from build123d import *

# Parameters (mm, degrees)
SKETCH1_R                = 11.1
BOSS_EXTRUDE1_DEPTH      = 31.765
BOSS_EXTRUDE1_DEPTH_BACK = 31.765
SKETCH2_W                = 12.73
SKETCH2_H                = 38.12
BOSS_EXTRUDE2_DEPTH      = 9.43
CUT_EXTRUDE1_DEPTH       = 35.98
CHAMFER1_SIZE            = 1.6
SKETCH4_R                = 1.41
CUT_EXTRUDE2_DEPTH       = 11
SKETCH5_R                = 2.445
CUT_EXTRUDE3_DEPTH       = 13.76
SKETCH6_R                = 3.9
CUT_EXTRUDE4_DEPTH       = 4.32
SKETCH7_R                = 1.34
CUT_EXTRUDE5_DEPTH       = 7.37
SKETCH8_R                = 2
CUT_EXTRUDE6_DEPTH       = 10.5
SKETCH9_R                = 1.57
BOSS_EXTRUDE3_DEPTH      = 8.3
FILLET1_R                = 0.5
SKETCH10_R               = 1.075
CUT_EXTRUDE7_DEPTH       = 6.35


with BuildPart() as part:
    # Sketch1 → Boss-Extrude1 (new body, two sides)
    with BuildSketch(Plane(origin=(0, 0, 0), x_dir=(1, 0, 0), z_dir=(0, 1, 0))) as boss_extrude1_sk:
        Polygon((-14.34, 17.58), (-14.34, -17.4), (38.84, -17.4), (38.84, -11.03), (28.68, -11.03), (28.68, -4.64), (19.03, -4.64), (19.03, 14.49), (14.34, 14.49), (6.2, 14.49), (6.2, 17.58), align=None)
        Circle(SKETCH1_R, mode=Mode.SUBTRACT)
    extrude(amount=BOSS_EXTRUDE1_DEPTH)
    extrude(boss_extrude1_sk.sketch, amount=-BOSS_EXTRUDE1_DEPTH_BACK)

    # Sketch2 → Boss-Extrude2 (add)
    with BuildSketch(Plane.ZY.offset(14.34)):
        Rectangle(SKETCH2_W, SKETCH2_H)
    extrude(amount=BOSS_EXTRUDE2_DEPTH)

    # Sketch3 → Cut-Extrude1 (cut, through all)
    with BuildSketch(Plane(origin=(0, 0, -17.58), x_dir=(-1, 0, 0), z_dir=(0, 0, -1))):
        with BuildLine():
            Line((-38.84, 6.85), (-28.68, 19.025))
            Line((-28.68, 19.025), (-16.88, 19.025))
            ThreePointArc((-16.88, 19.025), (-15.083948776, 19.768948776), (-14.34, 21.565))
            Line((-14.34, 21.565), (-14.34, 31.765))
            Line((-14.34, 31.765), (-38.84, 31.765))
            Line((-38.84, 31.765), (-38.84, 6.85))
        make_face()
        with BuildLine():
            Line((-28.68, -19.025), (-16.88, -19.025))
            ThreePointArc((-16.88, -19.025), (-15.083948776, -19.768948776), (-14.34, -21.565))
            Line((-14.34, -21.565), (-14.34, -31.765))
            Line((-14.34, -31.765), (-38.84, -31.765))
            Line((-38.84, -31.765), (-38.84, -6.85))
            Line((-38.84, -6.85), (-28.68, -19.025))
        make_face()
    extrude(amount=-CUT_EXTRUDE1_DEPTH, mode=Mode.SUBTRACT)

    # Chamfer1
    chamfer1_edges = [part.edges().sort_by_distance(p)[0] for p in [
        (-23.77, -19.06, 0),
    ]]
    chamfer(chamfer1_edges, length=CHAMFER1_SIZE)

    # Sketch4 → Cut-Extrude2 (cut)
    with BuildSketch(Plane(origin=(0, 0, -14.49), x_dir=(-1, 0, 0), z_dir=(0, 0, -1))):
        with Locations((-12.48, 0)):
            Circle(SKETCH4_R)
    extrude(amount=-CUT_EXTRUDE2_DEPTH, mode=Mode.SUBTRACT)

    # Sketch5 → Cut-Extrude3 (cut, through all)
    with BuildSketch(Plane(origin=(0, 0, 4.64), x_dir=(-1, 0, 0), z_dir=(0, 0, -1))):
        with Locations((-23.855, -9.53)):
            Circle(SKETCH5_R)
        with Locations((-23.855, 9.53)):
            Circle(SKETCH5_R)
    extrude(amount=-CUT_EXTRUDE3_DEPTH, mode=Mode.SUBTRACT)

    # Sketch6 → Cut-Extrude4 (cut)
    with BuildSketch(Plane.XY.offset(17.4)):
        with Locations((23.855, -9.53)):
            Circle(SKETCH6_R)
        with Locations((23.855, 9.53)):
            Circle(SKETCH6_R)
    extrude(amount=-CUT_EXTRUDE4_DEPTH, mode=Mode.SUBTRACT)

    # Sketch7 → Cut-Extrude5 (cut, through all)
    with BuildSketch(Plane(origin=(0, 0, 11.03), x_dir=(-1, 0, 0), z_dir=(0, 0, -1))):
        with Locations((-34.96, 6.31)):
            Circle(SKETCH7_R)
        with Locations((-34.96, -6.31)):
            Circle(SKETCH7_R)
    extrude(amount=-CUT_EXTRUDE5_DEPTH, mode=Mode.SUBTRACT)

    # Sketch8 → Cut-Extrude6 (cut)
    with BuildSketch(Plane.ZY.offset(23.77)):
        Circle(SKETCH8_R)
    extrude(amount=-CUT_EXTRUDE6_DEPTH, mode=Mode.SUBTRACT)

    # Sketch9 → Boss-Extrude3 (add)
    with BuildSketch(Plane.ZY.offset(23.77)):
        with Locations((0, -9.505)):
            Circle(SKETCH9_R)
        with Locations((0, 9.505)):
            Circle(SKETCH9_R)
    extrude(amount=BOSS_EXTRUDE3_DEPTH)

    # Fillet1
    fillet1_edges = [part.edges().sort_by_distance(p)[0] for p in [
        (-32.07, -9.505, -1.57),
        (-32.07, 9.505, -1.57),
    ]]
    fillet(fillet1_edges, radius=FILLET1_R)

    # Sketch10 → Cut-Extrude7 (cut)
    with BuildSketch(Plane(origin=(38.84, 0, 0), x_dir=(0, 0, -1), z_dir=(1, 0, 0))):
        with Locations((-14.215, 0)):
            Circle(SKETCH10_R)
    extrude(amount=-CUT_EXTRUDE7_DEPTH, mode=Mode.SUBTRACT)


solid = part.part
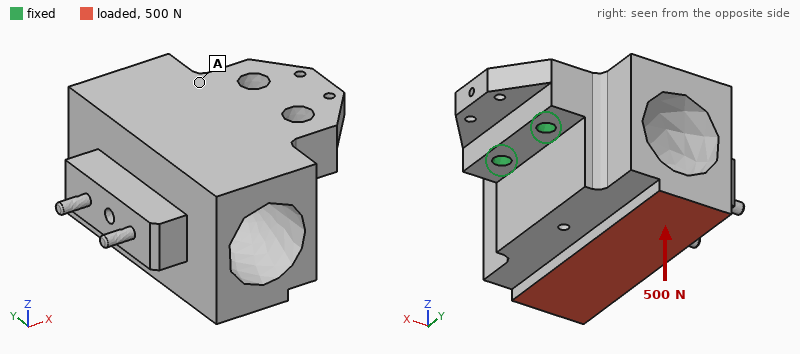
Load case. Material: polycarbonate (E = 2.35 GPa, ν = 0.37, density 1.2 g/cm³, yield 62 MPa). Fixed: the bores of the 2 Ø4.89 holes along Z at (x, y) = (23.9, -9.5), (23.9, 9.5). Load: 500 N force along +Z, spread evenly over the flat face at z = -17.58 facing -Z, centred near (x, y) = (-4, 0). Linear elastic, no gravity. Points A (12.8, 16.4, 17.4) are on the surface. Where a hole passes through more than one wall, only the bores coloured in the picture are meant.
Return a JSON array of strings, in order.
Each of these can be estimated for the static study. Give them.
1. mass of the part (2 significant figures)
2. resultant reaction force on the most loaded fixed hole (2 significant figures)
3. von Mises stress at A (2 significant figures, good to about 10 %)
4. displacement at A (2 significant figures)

["64 g", "250 N", "5.1 MPa", "0.19 mm"]
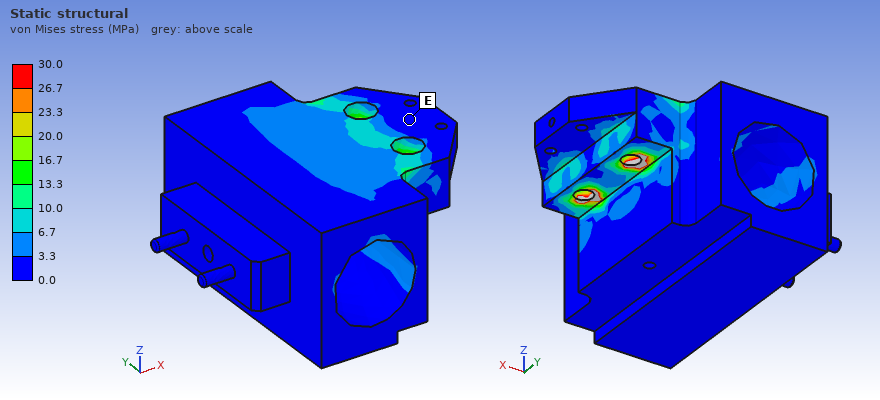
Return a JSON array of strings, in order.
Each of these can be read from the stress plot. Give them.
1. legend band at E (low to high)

["0.0 to 3.3 MPa"]
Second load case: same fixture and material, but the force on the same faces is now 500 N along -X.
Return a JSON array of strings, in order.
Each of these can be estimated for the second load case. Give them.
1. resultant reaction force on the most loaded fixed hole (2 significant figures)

["250 N"]
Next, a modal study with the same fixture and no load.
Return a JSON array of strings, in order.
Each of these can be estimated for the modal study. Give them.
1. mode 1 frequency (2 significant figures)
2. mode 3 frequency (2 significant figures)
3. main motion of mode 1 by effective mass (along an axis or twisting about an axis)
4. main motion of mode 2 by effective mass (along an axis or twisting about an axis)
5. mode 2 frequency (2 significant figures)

["600 Hz", "1700 Hz", "along Z", "along Y", "1200 Hz"]
